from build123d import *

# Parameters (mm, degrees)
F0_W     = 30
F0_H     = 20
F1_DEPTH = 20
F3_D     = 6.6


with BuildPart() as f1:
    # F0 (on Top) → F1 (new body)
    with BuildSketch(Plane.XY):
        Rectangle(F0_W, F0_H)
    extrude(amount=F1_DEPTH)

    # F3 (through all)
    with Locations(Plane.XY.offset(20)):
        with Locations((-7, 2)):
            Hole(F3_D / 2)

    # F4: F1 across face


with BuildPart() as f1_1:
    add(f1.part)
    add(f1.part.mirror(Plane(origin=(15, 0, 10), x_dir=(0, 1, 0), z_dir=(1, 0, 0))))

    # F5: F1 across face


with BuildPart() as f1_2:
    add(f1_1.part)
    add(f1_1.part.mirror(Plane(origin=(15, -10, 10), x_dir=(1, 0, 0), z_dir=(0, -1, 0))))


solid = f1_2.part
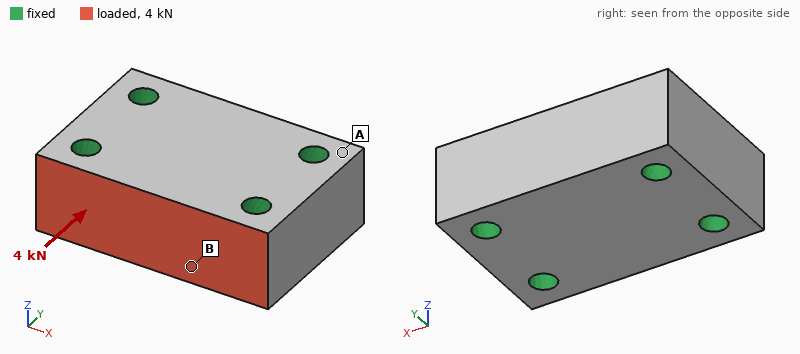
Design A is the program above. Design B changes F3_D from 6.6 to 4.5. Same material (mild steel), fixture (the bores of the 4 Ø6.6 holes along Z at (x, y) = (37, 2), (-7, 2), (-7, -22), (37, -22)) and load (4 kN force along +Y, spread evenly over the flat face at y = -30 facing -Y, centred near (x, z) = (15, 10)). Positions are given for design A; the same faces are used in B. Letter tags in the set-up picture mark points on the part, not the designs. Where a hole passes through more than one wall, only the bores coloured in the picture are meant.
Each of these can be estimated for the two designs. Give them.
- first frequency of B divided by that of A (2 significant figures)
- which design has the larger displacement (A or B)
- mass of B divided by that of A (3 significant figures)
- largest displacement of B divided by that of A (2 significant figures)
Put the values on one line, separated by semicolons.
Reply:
0.90; B; 1.03; 1.1
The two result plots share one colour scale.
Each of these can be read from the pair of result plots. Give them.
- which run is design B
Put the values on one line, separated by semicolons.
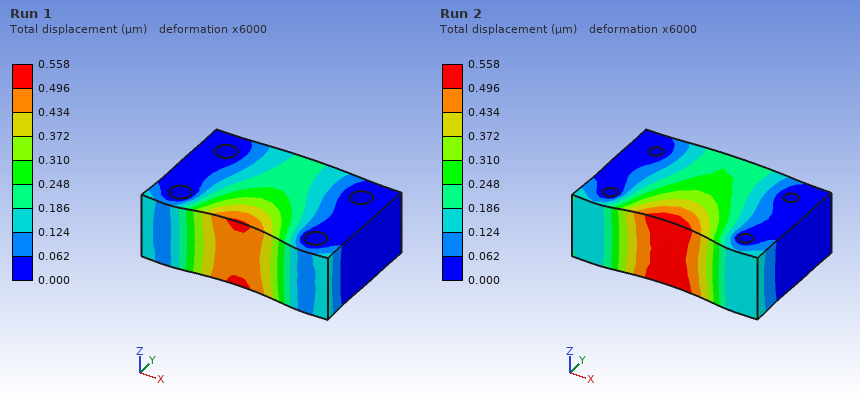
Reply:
Run 2
